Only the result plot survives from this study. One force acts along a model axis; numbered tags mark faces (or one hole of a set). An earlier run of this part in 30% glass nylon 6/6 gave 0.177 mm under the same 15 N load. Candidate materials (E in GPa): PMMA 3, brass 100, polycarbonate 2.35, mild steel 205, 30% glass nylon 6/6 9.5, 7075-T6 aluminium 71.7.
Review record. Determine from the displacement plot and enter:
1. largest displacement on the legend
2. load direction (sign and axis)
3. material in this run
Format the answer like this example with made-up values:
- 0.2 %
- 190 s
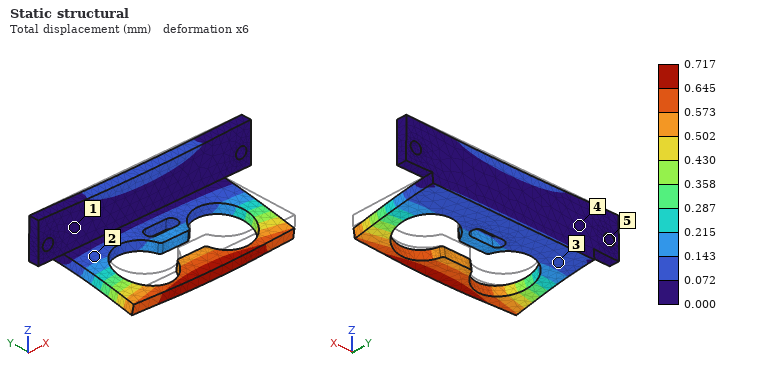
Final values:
- 0.717 mm
- -Z
- polycarbonate
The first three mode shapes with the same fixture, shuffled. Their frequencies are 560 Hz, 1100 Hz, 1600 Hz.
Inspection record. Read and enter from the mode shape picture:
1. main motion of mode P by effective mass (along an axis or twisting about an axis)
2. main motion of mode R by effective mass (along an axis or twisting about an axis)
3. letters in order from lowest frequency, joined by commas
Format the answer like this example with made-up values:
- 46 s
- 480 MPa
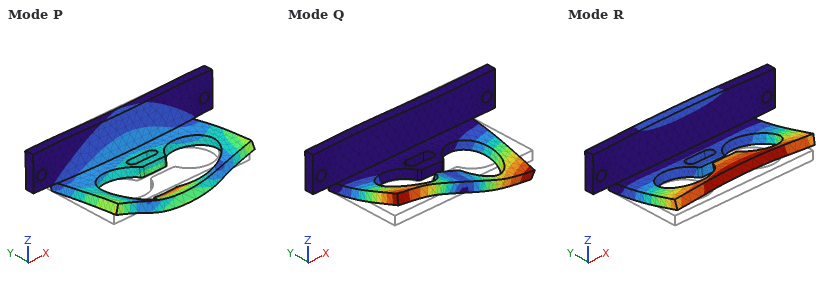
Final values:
- along Y
- along Z
- R, Q, P
